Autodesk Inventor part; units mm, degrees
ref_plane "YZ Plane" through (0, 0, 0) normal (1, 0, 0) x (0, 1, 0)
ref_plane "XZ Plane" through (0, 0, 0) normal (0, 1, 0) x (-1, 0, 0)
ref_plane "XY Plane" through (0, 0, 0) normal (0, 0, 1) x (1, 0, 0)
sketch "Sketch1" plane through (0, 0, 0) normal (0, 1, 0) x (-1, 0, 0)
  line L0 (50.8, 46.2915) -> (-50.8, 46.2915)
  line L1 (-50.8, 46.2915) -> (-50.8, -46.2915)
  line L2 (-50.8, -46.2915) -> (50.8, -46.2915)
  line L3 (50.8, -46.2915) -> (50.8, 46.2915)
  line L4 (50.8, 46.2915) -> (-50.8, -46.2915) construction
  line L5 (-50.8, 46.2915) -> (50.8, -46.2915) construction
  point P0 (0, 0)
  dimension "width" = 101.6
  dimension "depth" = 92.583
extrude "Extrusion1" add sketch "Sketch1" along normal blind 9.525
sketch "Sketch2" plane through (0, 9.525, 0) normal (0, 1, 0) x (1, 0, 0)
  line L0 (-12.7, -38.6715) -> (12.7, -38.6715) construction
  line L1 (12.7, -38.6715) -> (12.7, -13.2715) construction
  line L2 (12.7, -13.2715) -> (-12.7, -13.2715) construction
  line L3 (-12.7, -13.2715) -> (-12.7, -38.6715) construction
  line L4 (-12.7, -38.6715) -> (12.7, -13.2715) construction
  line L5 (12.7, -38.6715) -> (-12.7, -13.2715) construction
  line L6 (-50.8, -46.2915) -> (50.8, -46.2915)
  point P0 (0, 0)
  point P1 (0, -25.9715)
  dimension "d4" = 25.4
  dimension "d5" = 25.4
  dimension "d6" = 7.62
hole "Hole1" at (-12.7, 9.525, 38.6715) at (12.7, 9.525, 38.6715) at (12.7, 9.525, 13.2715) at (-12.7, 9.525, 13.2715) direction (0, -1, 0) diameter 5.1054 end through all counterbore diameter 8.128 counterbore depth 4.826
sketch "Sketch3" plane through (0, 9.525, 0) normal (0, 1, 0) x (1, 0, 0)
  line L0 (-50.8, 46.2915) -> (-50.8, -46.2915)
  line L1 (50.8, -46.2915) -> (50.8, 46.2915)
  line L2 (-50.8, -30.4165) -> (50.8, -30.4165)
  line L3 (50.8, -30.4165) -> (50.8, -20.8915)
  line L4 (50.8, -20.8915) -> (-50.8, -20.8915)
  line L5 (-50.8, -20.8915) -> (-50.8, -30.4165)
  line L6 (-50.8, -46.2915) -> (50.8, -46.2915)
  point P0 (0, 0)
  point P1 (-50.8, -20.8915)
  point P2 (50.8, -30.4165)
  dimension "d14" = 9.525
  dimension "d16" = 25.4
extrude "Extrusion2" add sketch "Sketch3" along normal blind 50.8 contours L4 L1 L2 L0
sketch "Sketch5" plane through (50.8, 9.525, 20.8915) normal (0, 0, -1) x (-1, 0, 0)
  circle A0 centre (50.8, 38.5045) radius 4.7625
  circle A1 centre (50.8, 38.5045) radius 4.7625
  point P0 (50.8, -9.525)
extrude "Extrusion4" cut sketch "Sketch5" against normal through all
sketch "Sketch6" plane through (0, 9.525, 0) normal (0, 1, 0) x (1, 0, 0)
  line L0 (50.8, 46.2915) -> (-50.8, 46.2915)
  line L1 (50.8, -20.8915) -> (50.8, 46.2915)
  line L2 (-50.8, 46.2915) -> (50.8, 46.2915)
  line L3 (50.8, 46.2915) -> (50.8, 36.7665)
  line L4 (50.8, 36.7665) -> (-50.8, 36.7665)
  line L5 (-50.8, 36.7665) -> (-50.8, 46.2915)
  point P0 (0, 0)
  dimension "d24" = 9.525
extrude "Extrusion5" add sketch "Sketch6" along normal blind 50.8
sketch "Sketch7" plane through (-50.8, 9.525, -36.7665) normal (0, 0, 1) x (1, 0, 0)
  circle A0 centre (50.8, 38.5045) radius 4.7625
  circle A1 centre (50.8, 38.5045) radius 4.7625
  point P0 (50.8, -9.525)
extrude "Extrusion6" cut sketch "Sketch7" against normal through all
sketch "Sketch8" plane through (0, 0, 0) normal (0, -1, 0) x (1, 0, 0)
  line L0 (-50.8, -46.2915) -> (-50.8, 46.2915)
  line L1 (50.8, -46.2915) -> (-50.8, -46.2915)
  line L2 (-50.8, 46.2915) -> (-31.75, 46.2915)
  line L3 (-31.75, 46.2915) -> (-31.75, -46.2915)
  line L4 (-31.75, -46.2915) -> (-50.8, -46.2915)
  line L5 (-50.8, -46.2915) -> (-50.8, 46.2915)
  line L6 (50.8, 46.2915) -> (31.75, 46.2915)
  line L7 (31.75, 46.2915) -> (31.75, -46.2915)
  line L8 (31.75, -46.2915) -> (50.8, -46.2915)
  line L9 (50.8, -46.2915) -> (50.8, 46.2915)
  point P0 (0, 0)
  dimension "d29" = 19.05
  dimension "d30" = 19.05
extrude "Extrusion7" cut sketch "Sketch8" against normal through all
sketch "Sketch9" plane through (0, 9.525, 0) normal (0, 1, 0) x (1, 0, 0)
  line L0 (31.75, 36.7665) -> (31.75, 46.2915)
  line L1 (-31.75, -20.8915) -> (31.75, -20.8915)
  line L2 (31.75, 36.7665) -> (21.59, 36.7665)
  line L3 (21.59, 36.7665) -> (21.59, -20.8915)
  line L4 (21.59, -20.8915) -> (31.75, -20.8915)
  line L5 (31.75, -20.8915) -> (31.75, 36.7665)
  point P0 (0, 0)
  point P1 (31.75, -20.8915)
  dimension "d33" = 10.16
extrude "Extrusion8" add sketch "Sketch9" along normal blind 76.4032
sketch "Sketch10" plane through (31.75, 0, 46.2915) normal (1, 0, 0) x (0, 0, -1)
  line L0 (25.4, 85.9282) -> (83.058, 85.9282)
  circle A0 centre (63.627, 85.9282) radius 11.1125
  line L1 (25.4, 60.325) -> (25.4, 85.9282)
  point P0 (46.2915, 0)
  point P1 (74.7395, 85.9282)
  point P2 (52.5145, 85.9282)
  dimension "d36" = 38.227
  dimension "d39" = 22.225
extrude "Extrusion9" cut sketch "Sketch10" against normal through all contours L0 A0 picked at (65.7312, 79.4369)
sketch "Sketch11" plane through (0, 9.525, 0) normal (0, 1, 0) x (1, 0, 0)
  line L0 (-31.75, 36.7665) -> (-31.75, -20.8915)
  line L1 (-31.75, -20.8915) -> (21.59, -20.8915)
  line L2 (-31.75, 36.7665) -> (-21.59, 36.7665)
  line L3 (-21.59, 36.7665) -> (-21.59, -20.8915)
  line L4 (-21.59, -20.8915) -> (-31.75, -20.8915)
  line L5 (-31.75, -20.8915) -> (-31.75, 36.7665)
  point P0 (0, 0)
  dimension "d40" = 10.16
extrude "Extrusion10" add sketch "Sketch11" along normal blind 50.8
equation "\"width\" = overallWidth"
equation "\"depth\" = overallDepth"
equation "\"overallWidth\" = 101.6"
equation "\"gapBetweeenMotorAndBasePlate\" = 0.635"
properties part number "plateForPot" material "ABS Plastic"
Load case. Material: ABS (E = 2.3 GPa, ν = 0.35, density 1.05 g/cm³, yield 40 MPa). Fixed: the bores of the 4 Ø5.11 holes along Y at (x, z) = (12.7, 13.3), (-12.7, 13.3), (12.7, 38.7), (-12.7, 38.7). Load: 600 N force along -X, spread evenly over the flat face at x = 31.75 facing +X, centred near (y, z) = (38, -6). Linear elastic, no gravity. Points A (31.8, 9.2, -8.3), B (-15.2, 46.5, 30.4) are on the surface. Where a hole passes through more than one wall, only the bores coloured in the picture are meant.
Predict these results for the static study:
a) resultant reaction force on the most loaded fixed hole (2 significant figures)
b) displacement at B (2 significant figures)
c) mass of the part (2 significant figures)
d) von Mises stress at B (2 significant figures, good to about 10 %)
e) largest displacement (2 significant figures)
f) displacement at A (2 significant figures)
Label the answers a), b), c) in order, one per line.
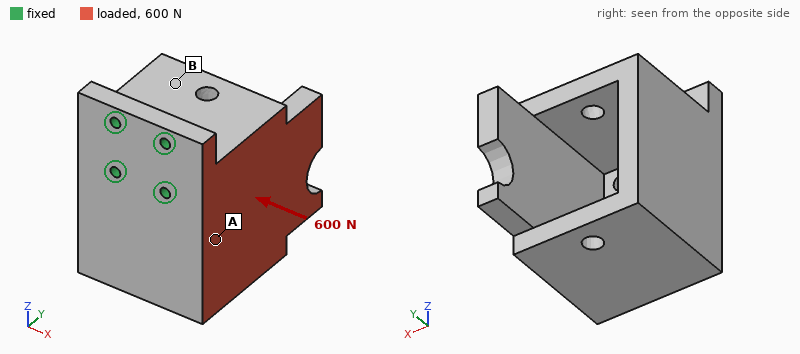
a) 600 N
b) 0.19 mm
c) 200 g
d) 1.8 MPa
e) 0.75 mm
f) 0.17 mm
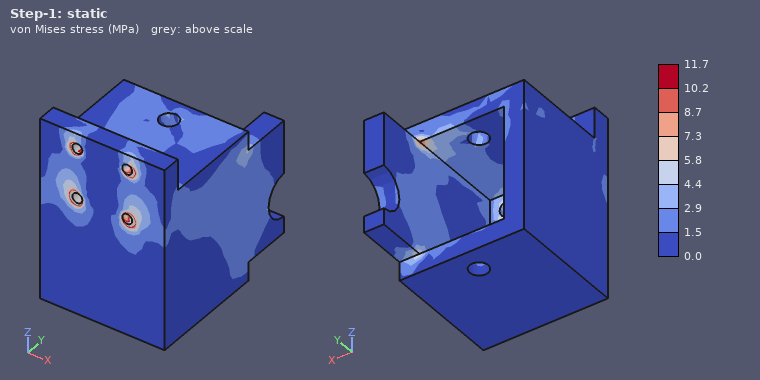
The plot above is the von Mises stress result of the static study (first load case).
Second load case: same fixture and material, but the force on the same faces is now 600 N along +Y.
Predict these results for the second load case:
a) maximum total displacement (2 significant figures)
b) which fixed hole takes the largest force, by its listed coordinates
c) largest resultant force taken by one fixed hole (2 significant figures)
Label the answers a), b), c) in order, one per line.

a) 0.85 mm
b) (12.7, 13.3)
c) 970 N
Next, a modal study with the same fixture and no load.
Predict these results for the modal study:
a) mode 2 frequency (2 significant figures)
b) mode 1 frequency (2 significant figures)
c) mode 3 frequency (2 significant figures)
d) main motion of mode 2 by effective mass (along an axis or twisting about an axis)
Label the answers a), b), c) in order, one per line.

a) 550 Hz
b) 400 Hz
c) 1100 Hz
d) along X
